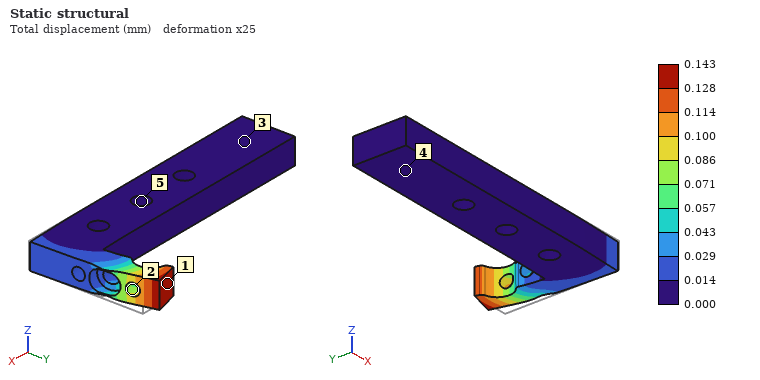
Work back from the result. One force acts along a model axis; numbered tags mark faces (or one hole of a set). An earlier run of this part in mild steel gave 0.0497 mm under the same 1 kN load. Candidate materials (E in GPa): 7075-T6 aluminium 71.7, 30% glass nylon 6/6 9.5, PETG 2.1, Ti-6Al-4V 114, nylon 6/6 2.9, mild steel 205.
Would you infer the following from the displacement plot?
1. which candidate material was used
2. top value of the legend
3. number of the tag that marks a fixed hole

7075-T6 aluminium
0.143 mm
5
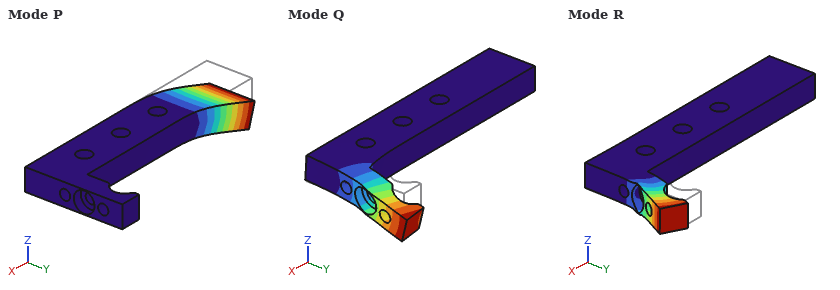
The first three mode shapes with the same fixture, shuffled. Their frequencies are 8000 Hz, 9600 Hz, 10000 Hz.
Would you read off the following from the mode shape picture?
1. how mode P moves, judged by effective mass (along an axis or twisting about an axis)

along Z
